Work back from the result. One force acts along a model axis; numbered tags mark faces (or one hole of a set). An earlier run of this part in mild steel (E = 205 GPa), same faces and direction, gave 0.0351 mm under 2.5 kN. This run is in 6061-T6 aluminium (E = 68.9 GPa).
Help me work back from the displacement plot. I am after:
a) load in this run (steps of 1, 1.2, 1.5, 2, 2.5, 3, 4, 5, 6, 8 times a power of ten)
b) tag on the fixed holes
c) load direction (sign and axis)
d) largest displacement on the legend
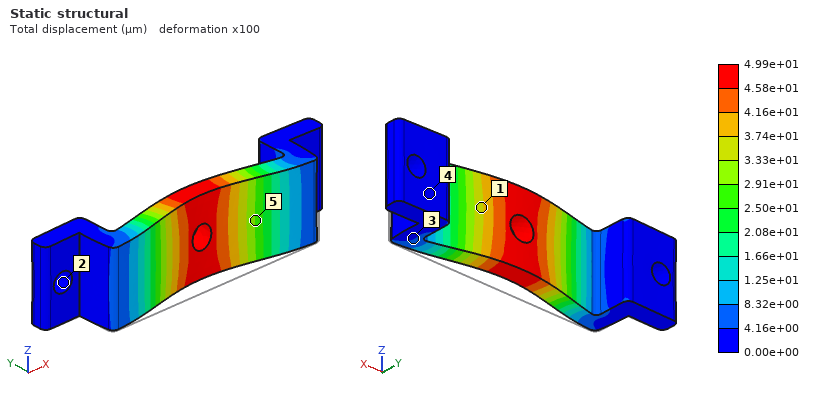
1.2 kN
2
+Y
4.99e+01 µm
